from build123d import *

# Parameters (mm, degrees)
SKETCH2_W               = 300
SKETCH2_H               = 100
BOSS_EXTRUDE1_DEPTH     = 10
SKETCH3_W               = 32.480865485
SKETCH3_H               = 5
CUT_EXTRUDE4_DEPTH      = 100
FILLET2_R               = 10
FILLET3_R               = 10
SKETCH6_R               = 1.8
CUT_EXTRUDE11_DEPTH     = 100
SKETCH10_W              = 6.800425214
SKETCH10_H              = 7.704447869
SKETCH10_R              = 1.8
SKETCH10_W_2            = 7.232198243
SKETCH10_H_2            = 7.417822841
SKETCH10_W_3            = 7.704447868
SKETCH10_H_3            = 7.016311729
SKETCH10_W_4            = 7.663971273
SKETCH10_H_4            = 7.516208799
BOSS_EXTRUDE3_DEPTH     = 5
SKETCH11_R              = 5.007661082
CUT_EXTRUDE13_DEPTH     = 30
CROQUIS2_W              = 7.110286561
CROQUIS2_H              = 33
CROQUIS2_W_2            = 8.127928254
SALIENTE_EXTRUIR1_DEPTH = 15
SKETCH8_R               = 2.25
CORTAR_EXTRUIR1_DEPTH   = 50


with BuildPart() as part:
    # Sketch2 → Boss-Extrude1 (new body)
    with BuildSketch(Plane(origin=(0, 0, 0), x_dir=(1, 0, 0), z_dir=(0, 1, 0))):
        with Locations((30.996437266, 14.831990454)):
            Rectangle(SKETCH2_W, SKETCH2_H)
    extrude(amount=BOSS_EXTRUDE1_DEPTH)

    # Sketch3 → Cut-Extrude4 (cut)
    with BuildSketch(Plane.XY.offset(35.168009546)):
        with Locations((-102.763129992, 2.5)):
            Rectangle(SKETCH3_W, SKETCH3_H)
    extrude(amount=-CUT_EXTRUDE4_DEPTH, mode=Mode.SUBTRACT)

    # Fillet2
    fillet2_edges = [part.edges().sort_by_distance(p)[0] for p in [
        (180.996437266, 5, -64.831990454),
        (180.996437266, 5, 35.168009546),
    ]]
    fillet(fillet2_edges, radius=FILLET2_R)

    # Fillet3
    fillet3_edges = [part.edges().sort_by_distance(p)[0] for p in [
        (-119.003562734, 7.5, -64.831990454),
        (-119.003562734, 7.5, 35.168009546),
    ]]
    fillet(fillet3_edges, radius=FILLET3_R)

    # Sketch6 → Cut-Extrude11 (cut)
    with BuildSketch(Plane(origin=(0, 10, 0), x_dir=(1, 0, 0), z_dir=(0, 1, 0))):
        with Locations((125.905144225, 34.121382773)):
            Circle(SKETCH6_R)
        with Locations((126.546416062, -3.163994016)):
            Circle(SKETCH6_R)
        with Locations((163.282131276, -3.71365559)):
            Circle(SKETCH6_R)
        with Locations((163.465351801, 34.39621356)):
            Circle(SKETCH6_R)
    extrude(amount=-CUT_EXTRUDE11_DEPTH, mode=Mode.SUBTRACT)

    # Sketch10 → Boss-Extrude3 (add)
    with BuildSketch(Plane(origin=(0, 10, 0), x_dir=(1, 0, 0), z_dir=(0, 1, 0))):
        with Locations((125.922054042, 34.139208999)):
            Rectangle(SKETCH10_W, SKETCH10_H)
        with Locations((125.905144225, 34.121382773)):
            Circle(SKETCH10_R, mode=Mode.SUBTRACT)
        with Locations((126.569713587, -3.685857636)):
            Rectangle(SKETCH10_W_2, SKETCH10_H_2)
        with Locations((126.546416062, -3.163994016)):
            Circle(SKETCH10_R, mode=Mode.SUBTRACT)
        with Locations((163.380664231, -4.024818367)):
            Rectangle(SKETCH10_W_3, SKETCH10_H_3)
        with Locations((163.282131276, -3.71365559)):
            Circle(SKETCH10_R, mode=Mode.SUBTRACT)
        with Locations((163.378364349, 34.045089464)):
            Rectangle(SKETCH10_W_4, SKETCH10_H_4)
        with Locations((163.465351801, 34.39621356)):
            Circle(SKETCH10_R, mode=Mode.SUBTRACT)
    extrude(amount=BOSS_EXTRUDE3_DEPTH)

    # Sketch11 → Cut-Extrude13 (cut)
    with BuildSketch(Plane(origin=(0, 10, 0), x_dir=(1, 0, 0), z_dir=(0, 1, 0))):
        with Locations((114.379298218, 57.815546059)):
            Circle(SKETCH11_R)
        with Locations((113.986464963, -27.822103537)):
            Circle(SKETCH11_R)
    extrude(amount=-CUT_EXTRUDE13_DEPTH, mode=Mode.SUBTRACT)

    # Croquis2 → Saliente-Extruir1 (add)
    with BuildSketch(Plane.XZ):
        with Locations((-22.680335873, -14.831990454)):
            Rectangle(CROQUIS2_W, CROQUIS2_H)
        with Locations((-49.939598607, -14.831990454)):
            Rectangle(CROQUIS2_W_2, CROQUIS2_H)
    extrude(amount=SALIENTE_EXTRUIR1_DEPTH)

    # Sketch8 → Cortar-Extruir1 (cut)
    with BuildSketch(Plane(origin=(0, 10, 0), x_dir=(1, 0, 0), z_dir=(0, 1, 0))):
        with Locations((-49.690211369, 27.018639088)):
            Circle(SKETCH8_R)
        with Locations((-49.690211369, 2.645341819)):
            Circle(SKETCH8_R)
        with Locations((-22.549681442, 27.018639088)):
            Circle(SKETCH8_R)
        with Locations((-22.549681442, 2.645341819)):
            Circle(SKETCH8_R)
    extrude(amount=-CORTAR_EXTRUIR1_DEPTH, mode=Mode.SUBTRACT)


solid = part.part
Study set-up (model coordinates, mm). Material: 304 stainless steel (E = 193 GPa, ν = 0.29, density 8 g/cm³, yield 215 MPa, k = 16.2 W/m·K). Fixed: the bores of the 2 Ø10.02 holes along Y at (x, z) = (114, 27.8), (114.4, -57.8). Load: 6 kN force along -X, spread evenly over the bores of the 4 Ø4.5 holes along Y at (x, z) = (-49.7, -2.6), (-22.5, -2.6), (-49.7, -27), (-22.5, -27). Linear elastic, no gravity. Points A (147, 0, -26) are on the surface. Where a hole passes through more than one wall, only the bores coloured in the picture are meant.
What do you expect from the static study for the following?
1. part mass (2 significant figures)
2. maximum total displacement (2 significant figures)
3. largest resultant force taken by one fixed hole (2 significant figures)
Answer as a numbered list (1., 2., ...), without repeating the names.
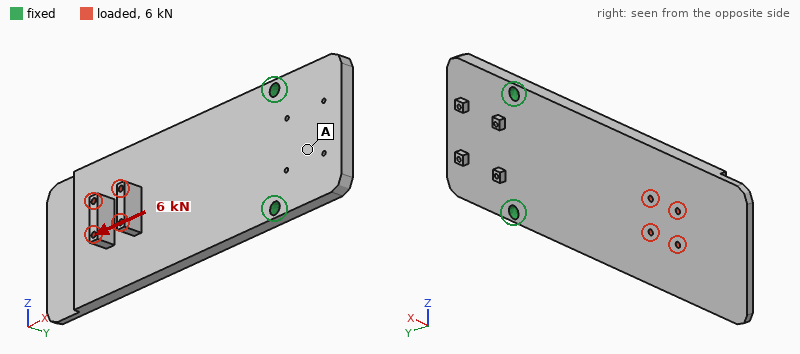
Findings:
1. 2.3 kg
2. 0.69 mm
3. 3.0 kN
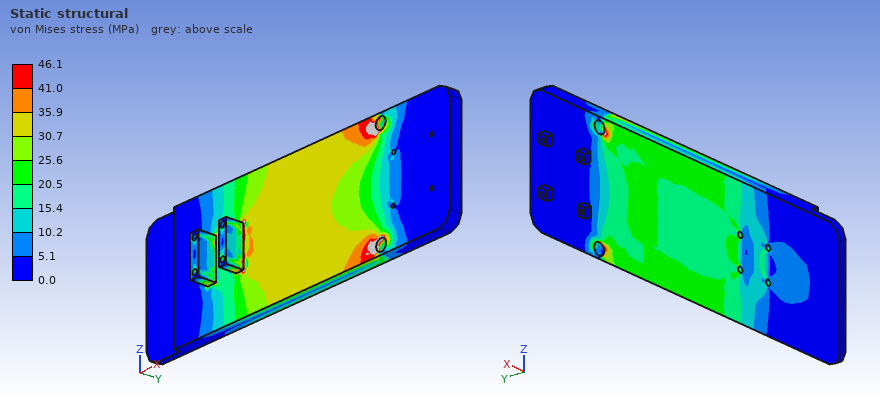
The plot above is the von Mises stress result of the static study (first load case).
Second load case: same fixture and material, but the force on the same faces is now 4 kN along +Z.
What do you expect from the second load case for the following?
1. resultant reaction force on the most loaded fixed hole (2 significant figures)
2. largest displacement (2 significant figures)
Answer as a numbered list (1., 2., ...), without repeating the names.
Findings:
1. 7.2 kN
2. 0.10 mm
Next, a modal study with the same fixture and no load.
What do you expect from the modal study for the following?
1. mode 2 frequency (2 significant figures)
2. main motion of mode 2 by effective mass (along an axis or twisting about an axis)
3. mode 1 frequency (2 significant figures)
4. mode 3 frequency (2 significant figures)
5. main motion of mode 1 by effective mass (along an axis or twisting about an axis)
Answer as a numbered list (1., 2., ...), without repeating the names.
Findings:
1. 770 Hz
2. twisting about X
3. 160 Hz
4. 950 Hz
5. along Y
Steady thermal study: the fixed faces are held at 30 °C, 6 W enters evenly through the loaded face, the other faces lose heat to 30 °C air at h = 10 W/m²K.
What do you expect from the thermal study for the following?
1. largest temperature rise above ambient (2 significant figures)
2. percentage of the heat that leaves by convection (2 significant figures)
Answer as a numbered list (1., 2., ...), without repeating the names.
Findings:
1. 22 K
2. 84 %
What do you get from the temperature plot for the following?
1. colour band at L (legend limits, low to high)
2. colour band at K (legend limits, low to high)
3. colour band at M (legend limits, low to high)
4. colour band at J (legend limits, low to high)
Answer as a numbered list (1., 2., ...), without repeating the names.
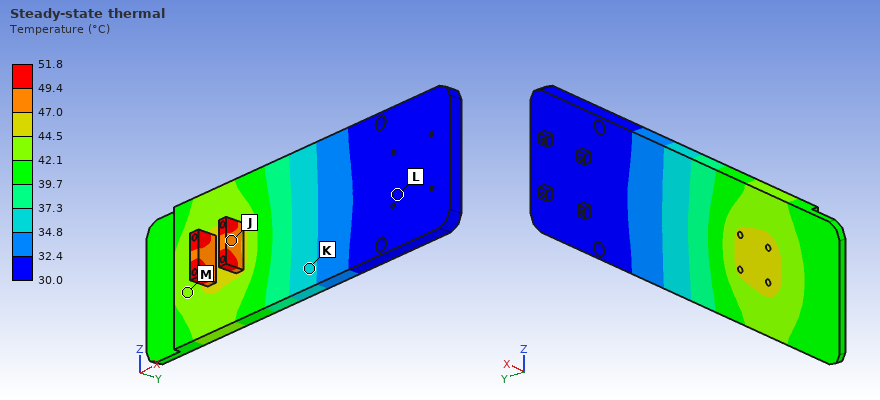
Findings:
1. 30.0 to 32.4 °C
2. 34.8 to 37.3 °C
3. 42.1 to 44.5 °C
4. 47.0 to 49.4 °C
